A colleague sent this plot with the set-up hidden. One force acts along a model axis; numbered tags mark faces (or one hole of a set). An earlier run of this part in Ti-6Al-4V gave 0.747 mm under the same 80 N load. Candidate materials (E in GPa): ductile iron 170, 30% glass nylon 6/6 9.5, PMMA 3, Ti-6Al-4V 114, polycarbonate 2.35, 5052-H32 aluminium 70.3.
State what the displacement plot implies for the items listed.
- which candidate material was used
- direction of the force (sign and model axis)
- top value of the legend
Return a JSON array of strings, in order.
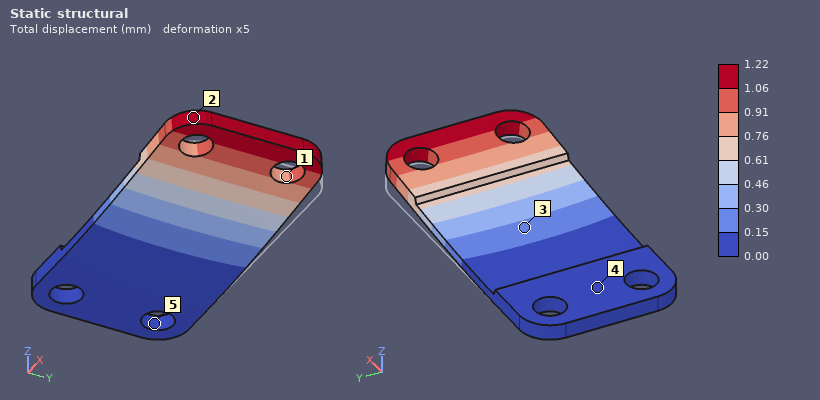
["5052-H32 aluminium", "+Z", "1.22 mm"]
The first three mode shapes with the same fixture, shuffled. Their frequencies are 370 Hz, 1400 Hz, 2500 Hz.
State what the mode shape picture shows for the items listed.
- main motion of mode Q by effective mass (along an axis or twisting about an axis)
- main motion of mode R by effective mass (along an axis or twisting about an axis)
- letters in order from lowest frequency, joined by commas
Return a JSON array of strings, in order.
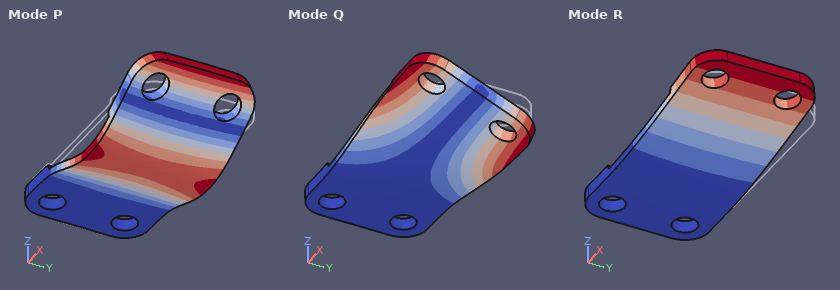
["twisting about X", "along Z", "R, Q, P"]
